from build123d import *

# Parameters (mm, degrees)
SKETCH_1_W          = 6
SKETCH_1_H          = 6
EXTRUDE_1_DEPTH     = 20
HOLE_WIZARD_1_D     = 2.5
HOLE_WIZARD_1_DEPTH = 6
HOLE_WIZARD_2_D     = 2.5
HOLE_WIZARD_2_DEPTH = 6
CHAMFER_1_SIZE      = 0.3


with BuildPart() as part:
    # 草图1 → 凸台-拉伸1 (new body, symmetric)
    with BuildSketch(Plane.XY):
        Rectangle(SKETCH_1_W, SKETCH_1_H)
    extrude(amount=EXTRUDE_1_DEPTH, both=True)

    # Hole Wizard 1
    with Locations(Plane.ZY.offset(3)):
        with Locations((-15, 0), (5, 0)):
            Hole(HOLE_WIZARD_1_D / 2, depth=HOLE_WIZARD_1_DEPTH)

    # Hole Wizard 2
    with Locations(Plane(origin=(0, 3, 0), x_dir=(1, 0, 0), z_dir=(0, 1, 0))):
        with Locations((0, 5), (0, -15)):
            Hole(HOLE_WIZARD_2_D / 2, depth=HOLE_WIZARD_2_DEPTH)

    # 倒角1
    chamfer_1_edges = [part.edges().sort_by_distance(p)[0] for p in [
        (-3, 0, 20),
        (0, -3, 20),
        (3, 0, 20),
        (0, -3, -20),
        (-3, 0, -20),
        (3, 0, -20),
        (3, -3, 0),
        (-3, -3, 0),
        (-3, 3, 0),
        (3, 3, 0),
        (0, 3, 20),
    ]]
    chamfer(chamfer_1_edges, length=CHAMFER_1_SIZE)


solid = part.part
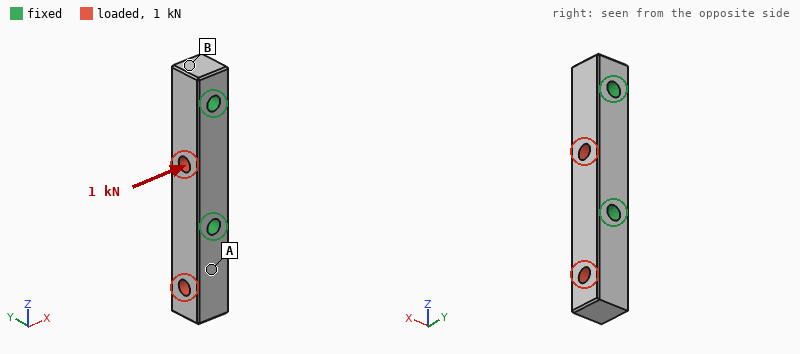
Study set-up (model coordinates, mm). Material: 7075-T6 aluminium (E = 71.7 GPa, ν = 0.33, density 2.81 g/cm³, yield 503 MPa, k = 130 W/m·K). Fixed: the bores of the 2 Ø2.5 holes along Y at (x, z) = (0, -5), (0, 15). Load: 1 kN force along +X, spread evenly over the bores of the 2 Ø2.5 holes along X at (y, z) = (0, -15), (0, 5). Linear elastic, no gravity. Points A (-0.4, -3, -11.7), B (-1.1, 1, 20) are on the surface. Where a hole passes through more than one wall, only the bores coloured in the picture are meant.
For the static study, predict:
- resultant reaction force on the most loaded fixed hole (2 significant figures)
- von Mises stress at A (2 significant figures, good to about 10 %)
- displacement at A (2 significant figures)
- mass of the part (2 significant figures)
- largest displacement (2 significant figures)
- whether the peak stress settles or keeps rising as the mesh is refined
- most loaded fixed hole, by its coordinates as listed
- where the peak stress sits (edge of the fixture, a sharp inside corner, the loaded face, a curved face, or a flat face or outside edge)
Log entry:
810 N
39 MPa
17 µm
3.7 g
52 µm
keeps rising
(0, -5)
edge of the fixture
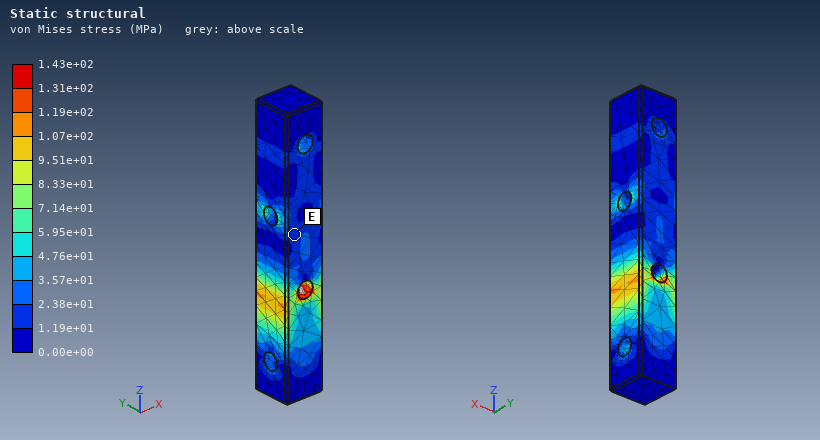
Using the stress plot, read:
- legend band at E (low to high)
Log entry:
1.19e+01 to 2.38e+01 MPa
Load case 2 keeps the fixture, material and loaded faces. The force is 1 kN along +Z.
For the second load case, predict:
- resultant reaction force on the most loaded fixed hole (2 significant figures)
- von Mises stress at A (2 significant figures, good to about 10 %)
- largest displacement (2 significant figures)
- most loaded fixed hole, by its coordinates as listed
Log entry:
740 N
15 MPa
2.6 µm
(0, -5)
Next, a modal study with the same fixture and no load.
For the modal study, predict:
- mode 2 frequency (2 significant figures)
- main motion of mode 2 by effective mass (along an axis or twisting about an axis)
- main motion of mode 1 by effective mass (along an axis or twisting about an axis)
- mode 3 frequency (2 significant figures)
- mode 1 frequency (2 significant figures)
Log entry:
21 kHz
along Y
along X
49 kHz
18 kHz
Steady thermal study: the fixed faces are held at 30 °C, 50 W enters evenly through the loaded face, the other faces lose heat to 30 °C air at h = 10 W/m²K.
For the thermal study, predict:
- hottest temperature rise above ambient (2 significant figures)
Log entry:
59 K
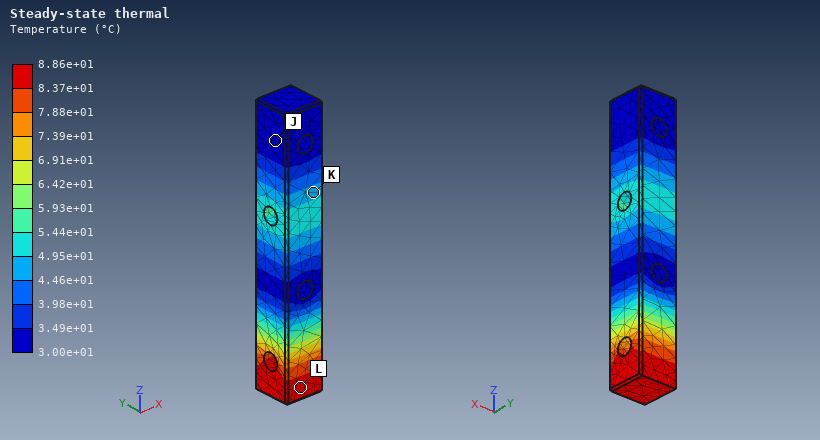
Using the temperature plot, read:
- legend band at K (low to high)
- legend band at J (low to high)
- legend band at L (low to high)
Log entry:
4.46e+01 to 4.95e+01 °C
3.00e+01 to 3.49e+01 °C
8.37e+01 to 8.86e+01 °C
